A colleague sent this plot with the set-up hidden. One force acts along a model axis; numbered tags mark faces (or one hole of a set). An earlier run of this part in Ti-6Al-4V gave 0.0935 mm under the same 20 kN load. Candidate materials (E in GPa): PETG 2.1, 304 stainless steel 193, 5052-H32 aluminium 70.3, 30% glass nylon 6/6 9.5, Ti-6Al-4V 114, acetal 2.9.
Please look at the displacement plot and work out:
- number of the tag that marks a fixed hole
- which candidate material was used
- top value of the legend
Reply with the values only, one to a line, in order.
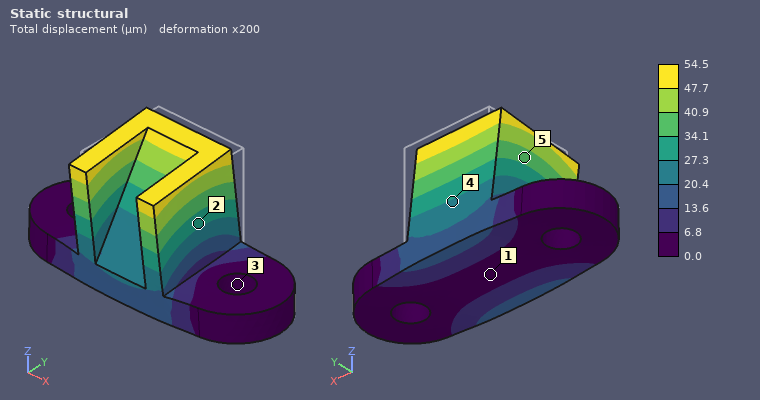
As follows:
3
304 stainless steel
54.5 µm
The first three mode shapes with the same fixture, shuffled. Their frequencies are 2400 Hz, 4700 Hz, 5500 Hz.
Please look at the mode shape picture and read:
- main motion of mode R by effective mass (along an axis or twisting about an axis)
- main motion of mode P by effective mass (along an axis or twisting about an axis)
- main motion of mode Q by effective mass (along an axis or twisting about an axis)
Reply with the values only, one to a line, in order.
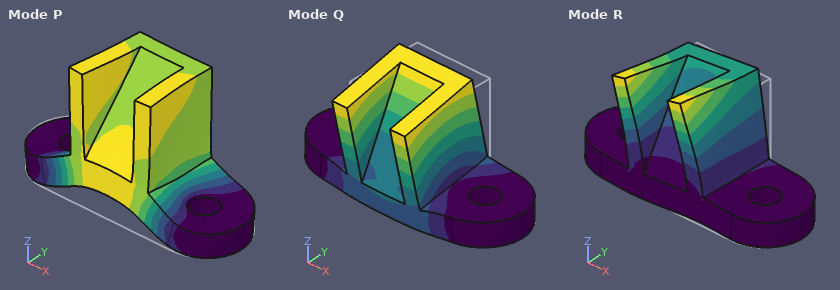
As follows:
along X
along Z
along Y
